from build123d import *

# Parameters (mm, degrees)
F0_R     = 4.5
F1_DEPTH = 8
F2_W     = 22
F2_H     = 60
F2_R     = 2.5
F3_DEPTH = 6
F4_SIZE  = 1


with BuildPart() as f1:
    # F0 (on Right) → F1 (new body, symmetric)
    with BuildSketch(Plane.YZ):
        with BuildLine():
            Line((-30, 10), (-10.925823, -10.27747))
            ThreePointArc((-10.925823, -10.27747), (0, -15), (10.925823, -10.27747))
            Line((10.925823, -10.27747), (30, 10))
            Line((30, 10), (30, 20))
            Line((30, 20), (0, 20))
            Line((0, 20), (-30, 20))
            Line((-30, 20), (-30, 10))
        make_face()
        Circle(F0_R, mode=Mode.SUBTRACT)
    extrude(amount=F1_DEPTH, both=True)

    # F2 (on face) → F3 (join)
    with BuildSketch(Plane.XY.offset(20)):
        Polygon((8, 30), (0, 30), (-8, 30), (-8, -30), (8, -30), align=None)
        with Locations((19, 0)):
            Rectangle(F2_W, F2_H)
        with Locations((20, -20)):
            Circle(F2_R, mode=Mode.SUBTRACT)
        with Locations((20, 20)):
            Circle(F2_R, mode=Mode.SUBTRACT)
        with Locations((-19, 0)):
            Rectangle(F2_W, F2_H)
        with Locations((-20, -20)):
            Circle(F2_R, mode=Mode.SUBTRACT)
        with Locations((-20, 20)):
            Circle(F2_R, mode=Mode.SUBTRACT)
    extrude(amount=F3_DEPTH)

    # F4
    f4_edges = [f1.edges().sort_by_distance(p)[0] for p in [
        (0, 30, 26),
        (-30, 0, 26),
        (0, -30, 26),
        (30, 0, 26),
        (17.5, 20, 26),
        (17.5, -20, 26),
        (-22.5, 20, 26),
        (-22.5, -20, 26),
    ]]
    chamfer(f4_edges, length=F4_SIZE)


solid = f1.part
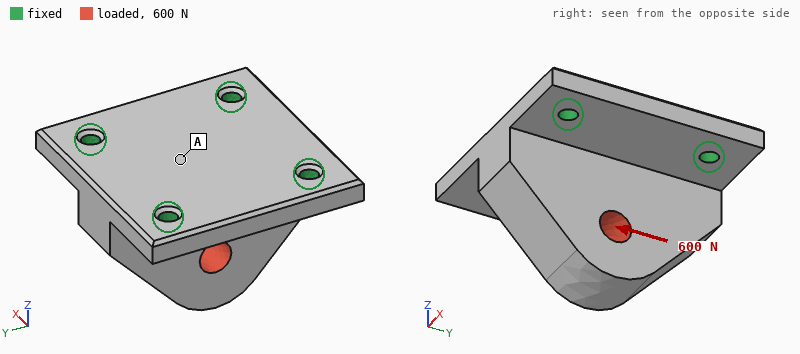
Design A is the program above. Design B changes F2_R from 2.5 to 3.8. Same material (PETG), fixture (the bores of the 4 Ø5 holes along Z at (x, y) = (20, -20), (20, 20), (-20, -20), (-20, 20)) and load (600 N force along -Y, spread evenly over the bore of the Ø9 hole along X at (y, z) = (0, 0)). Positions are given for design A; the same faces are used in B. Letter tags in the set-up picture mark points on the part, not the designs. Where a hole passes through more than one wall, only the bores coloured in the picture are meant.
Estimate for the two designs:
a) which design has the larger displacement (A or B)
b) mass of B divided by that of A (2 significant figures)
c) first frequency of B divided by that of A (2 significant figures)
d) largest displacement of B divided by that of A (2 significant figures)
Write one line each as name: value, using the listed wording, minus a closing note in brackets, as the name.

which design has the larger displacement: A
mass of B divided by that of A: 0.99
first frequency of B divided by that of A: 1.1
largest displacement of B divided by that of A: 0.79
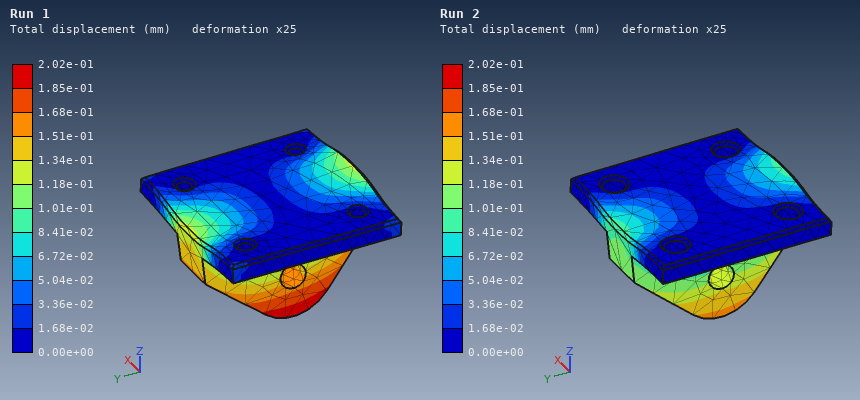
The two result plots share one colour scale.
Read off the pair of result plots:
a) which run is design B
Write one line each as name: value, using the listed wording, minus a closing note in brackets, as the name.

which run is design B: Run 2
